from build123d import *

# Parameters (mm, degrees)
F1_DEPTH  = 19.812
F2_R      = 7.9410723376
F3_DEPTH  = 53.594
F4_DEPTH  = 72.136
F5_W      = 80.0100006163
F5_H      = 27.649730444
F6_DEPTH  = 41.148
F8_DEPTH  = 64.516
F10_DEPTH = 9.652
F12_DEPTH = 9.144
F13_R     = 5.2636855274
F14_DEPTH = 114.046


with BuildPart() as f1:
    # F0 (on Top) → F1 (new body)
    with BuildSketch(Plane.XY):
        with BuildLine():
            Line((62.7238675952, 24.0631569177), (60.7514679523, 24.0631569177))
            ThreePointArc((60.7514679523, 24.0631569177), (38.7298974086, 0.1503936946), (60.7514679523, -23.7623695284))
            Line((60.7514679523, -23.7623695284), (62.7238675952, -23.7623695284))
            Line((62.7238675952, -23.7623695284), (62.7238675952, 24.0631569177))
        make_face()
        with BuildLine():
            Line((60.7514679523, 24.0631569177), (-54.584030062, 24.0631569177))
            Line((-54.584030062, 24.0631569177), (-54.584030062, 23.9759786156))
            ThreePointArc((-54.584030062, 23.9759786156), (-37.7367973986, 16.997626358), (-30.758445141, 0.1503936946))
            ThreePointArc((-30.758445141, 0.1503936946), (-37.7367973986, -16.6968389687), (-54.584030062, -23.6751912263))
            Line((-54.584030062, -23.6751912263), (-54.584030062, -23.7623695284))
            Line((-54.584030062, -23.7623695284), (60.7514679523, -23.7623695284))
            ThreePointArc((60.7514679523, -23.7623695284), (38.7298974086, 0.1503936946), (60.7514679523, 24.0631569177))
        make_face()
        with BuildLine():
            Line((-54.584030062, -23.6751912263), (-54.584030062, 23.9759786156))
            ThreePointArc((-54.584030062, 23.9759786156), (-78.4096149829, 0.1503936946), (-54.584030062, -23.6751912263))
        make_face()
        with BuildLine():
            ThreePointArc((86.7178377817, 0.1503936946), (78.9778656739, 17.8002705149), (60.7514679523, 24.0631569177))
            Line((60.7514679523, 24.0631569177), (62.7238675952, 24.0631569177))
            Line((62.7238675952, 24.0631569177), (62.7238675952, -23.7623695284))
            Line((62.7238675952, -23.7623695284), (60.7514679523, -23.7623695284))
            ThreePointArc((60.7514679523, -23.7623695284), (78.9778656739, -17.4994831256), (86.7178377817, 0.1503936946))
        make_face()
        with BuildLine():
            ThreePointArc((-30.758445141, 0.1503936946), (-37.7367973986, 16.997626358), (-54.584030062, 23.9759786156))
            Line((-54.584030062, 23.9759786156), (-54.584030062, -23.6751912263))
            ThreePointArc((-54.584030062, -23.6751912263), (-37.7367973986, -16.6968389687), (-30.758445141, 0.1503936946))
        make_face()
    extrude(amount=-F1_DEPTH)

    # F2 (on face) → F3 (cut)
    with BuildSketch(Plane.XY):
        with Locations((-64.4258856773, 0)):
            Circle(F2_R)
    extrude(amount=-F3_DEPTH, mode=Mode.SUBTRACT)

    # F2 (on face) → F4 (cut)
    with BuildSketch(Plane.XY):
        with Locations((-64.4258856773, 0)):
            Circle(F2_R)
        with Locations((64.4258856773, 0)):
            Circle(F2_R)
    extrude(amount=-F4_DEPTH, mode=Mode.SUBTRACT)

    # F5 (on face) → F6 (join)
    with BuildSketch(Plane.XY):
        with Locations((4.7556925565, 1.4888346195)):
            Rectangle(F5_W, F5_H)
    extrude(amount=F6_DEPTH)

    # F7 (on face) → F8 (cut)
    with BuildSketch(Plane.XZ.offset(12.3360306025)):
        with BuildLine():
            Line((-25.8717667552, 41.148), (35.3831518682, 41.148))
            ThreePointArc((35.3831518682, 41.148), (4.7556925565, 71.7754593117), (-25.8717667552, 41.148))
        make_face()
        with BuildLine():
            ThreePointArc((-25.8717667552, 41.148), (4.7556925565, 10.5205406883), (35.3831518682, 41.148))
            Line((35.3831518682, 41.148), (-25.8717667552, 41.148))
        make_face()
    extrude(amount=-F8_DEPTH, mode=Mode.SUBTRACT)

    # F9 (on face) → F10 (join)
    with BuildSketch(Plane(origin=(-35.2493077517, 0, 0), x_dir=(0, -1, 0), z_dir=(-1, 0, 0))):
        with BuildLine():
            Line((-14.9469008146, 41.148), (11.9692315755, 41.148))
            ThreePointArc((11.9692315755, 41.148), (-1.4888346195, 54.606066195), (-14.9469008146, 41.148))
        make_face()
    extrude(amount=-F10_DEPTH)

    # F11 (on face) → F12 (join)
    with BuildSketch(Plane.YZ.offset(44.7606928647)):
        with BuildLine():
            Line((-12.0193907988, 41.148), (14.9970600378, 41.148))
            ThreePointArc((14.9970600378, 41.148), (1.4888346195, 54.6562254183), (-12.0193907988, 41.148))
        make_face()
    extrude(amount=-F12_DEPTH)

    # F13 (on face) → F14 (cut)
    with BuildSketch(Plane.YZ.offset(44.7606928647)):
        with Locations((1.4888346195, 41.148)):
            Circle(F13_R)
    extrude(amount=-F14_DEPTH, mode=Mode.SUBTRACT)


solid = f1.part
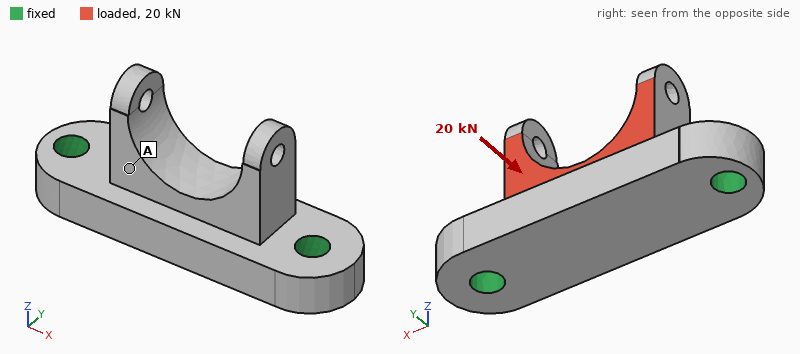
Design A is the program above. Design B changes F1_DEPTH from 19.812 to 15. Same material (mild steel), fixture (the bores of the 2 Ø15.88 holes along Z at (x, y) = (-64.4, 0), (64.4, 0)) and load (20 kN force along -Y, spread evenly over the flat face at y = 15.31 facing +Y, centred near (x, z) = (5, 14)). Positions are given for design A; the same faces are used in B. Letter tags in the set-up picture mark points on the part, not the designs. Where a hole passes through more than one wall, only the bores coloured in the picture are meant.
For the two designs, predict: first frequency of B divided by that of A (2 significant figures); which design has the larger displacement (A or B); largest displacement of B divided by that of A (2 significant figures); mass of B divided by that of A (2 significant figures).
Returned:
0.84
B
1.4
0.83
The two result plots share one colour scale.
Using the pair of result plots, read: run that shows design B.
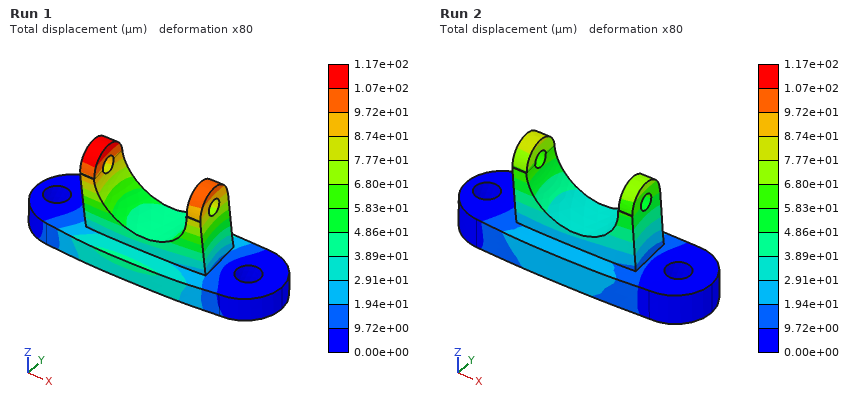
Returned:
Run 1
